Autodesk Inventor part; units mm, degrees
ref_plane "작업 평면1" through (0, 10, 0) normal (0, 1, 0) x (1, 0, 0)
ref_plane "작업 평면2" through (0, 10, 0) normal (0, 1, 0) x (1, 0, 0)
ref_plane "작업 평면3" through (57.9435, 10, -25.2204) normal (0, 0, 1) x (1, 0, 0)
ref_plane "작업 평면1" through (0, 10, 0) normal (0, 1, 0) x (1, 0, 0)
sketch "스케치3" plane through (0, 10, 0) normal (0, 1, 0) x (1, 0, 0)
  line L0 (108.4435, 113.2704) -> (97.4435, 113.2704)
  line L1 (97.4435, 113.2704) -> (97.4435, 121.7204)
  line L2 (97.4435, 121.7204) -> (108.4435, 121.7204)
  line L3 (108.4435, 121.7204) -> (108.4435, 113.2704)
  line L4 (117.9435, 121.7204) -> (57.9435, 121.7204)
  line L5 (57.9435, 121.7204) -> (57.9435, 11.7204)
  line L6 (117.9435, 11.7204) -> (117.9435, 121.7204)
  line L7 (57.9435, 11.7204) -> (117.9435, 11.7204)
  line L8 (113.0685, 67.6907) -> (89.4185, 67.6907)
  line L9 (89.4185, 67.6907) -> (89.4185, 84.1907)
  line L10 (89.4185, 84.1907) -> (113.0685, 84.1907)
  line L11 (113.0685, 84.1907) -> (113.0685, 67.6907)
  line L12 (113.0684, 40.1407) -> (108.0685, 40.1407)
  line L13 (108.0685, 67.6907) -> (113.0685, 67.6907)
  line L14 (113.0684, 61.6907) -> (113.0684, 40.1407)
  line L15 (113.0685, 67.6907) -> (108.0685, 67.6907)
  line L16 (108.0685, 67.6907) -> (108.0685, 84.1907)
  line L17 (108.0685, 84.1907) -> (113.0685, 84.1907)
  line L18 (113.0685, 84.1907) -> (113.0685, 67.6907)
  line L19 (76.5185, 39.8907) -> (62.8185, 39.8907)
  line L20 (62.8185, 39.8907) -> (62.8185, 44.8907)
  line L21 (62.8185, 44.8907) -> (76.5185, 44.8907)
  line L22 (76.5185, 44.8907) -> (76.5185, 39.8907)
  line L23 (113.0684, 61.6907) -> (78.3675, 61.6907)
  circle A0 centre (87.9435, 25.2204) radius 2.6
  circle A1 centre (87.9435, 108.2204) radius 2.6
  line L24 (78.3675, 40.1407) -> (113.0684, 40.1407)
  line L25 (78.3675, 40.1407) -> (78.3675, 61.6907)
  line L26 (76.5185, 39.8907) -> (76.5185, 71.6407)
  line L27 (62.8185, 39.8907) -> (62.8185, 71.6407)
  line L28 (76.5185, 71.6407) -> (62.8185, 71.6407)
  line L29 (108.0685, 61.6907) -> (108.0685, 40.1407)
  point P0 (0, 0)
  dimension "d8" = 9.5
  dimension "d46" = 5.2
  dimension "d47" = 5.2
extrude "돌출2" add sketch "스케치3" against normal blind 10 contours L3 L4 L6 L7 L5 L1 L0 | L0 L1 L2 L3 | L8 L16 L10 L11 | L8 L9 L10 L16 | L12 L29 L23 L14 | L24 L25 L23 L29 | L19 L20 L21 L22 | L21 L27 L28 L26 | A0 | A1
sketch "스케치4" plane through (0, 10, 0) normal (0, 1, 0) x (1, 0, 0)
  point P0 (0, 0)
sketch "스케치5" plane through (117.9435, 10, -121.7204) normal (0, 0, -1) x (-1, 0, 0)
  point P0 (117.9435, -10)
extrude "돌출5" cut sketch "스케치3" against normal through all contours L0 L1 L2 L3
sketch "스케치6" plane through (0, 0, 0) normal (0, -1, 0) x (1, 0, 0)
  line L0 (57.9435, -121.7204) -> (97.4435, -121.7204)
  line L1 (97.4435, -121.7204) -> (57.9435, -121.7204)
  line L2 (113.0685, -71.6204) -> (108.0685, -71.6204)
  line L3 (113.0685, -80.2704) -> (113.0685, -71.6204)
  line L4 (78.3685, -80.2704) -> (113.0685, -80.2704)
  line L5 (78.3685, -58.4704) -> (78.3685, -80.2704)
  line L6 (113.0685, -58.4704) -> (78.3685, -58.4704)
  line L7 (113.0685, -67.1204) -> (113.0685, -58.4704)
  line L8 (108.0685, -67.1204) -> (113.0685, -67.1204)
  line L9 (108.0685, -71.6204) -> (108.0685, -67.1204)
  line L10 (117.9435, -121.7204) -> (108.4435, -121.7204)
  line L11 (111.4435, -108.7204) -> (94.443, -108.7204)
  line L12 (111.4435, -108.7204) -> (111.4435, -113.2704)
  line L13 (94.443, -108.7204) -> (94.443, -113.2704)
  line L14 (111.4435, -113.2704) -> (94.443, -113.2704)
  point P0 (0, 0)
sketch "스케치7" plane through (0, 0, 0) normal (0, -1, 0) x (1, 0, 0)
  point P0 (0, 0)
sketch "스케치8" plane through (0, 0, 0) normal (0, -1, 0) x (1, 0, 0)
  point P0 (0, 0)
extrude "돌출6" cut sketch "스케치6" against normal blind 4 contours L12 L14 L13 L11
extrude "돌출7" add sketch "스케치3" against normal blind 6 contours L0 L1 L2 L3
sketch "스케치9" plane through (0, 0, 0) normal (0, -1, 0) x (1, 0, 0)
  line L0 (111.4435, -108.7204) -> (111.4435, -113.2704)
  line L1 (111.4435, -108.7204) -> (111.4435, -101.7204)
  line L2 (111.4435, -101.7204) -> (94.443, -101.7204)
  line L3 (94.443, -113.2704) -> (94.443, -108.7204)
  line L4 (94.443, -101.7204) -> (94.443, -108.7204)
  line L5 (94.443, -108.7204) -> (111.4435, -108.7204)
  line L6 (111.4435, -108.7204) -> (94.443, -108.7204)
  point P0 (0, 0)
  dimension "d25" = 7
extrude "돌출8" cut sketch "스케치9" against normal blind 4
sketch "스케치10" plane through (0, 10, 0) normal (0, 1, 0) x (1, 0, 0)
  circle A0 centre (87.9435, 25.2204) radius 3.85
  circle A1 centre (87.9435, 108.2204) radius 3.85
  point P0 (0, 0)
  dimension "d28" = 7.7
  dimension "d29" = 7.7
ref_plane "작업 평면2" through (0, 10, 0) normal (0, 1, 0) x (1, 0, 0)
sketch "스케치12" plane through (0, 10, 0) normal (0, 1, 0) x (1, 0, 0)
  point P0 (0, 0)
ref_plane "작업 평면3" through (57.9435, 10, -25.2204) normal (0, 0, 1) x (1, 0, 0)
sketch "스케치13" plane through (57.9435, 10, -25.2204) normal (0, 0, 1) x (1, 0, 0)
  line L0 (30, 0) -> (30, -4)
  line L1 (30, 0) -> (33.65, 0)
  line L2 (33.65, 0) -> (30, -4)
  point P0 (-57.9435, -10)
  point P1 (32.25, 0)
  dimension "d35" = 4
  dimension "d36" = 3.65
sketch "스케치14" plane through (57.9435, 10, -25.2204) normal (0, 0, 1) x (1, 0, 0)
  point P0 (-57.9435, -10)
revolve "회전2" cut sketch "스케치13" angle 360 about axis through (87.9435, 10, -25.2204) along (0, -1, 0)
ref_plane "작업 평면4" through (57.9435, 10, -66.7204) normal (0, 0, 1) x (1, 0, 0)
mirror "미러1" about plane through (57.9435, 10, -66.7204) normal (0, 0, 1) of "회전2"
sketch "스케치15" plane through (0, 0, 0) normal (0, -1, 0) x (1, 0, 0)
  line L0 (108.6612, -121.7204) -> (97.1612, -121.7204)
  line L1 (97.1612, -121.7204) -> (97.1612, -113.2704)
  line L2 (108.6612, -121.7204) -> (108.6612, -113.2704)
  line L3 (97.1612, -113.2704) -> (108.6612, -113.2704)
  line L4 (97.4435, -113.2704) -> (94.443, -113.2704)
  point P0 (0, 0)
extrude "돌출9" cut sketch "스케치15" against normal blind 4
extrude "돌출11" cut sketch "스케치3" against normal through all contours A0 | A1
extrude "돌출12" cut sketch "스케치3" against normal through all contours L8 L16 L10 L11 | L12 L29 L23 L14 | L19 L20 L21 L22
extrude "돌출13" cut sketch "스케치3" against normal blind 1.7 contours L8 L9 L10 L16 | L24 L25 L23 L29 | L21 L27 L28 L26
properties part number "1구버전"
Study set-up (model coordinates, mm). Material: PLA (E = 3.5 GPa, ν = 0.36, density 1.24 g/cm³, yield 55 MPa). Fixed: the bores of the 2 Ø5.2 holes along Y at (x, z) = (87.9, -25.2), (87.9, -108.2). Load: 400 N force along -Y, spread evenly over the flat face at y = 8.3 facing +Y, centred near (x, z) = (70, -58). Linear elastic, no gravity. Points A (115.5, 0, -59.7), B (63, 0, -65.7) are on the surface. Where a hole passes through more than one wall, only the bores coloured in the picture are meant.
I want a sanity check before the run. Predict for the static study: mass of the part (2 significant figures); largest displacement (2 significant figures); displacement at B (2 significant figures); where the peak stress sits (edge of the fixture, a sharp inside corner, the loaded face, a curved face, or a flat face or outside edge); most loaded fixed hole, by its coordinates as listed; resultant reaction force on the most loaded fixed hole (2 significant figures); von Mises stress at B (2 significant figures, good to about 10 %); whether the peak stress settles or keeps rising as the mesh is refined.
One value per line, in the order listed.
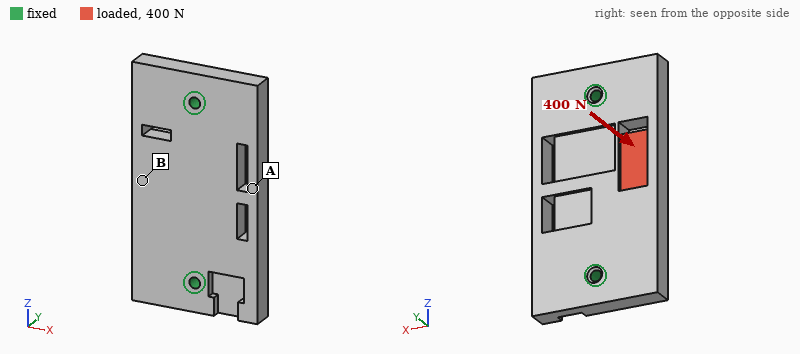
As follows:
74 g
0.38 mm
0.33 mm
edge of the fixture
(87.9, -25.2)
250 N
6.3 MPa
keeps rising
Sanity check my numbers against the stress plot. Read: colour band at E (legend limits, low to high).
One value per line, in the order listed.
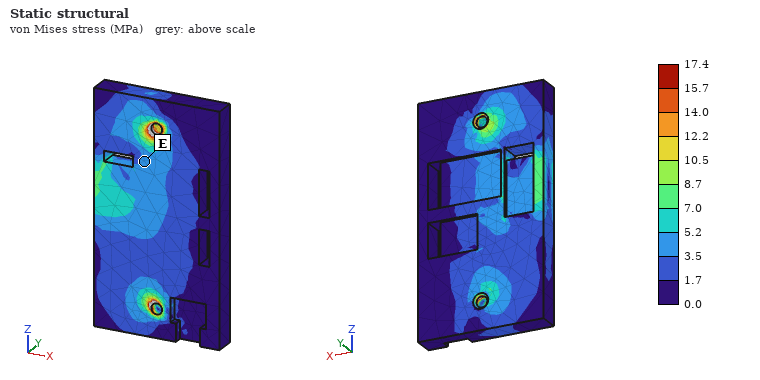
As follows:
3.5 to 5.2 MPa
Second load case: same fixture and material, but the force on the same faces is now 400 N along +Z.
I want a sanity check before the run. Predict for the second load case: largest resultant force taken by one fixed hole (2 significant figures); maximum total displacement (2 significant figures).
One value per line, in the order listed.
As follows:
220 N
28 µm
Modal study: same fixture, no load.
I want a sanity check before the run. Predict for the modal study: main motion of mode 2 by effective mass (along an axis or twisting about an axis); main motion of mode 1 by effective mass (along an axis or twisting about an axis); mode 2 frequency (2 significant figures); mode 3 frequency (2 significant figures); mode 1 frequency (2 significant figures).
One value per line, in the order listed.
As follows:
along Y
twisting about Z
1600 Hz
2300 Hz
1400 Hz
